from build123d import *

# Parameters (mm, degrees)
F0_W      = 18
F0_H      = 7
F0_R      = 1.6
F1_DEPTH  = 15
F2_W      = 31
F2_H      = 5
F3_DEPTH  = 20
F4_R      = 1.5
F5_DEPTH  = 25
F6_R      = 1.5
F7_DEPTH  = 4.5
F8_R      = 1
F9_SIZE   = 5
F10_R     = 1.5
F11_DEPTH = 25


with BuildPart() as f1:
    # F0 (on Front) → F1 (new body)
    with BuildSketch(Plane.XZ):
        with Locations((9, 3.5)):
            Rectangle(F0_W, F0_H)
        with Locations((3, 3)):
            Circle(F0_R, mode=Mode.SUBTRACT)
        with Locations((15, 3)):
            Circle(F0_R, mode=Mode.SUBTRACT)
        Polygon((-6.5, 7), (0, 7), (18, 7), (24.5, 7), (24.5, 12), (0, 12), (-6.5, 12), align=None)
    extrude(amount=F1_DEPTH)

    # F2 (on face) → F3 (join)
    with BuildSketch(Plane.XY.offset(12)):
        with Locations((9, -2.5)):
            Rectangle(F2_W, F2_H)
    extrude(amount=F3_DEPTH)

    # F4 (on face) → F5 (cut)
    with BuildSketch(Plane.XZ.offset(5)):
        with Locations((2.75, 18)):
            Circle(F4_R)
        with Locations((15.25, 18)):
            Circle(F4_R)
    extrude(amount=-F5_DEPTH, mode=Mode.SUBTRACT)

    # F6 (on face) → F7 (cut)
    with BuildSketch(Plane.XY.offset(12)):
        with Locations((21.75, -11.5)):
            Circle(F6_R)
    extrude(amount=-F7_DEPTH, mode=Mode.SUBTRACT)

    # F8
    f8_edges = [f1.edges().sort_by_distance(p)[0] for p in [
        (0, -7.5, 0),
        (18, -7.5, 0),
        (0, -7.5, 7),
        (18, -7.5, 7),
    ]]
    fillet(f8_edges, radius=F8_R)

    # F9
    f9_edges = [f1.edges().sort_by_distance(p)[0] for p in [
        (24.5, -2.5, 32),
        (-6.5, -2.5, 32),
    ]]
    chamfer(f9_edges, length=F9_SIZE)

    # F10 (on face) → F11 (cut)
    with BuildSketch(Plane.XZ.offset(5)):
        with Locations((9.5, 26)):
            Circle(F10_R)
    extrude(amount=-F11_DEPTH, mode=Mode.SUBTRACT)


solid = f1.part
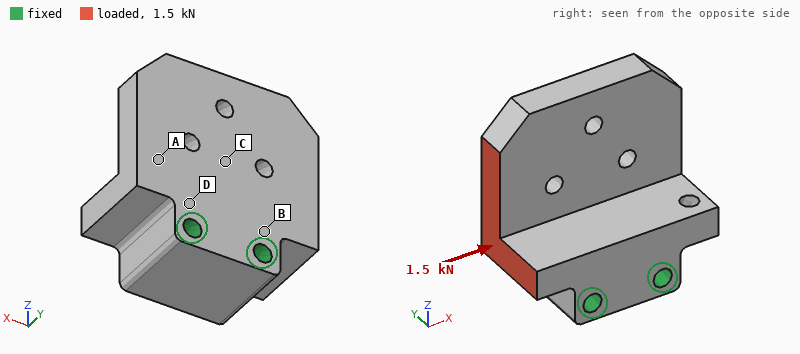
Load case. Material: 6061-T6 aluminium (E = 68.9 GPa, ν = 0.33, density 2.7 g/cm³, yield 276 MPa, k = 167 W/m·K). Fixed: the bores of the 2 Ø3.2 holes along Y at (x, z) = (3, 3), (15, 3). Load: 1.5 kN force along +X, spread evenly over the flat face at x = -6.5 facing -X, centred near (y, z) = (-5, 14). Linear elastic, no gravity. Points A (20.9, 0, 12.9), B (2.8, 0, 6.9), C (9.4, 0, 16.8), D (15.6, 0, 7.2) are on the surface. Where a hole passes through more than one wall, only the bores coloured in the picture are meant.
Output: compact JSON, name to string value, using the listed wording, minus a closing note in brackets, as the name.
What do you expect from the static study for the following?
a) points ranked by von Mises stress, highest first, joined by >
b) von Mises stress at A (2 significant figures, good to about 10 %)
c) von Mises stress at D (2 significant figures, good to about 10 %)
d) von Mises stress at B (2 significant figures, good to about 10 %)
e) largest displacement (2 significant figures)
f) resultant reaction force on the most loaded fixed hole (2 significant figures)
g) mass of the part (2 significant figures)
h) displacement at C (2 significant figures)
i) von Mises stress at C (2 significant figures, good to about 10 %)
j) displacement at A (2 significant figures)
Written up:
{"points ranked by von Mises stress, highest first, joined by >": "B > D > C > A", "von Mises stress at A": "4.2 MPa", "von Mises stress at D": "18 MPa", "von Mises stress at B": "25 MPa", "largest displacement": "15 µm", "resultant reaction force on the most loaded fixed hole": "1.5 kN", "mass of the part": "18 g", "displacement at C": "6.3 µm", "von Mises stress at C": "12 MPa", "displacement at A": "6.2 µm"}
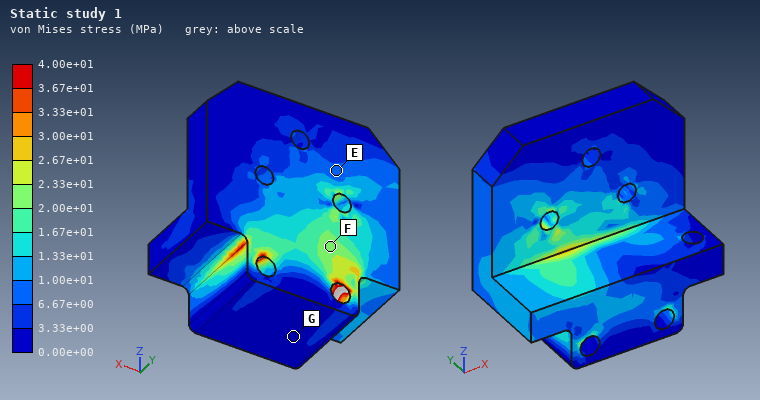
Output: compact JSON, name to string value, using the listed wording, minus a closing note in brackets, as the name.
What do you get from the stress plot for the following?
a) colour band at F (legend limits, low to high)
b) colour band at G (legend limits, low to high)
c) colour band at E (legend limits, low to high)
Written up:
{"colour band at F": "2.00e+01 to 2.33e+01 MPa", "colour band at G": "0.00e+00 to 3.33e+00 MPa", "colour band at E": "6.67e+00 to 1.00e+01 MPa"}
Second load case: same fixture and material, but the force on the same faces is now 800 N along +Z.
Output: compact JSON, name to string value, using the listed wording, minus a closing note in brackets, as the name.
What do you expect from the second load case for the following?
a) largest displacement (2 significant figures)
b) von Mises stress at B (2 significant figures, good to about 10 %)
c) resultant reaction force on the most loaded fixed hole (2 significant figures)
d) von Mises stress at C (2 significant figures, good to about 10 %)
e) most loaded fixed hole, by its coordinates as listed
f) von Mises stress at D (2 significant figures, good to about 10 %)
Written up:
{"largest displacement": "12 µm", "von Mises stress at B": "16 MPa", "resultant reaction force on the most loaded fixed hole": "1.3 kN", "von Mises stress at C": "6.3 MPa", "most loaded fixed hole, by its coordinates as listed": "(3, 3)", "von Mises stress at D": "8.0 MPa"}
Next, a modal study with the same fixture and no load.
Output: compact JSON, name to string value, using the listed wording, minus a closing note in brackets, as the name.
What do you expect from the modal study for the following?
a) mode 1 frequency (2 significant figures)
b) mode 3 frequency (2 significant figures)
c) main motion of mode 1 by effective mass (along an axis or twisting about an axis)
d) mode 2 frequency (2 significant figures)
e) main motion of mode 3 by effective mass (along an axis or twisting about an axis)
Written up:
{"mode 1 frequency": "7600 Hz", "mode 3 frequency": "15 kHz", "main motion of mode 1 by effective mass": "along Y", "mode 2 frequency": "14 kHz", "main motion of mode 3 by effective mass": "along X"}
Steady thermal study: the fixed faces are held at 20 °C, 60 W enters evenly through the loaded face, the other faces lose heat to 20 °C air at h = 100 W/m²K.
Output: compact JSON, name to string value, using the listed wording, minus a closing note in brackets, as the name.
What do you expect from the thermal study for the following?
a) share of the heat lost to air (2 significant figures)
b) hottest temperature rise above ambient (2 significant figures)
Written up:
{"share of the heat lost to air": "6.5 %", "hottest temperature rise above ambient": "41 K"}
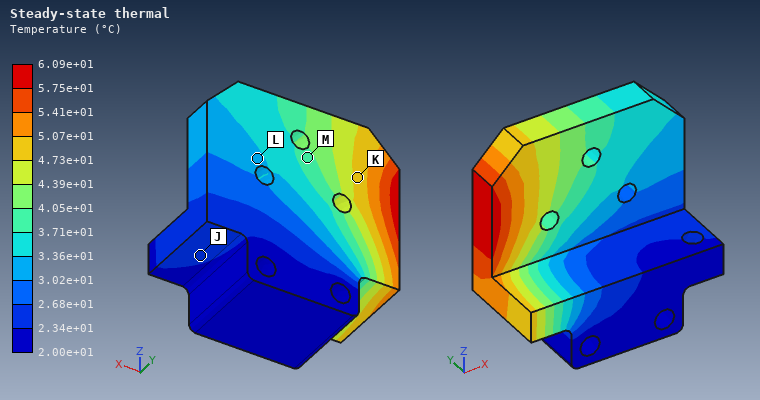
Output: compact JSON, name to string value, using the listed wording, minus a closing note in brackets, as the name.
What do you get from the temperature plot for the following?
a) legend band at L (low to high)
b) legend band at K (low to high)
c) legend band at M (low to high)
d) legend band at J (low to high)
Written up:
{"legend band at L": "3.02e+01 to 3.36e+01 °C", "legend band at K": "4.73e+01 to 5.07e+01 °C", "legend band at M": "3.71e+01 to 4.05e+01 °C", "legend band at J": "2.34e+01 to 2.68e+01 °C"}
